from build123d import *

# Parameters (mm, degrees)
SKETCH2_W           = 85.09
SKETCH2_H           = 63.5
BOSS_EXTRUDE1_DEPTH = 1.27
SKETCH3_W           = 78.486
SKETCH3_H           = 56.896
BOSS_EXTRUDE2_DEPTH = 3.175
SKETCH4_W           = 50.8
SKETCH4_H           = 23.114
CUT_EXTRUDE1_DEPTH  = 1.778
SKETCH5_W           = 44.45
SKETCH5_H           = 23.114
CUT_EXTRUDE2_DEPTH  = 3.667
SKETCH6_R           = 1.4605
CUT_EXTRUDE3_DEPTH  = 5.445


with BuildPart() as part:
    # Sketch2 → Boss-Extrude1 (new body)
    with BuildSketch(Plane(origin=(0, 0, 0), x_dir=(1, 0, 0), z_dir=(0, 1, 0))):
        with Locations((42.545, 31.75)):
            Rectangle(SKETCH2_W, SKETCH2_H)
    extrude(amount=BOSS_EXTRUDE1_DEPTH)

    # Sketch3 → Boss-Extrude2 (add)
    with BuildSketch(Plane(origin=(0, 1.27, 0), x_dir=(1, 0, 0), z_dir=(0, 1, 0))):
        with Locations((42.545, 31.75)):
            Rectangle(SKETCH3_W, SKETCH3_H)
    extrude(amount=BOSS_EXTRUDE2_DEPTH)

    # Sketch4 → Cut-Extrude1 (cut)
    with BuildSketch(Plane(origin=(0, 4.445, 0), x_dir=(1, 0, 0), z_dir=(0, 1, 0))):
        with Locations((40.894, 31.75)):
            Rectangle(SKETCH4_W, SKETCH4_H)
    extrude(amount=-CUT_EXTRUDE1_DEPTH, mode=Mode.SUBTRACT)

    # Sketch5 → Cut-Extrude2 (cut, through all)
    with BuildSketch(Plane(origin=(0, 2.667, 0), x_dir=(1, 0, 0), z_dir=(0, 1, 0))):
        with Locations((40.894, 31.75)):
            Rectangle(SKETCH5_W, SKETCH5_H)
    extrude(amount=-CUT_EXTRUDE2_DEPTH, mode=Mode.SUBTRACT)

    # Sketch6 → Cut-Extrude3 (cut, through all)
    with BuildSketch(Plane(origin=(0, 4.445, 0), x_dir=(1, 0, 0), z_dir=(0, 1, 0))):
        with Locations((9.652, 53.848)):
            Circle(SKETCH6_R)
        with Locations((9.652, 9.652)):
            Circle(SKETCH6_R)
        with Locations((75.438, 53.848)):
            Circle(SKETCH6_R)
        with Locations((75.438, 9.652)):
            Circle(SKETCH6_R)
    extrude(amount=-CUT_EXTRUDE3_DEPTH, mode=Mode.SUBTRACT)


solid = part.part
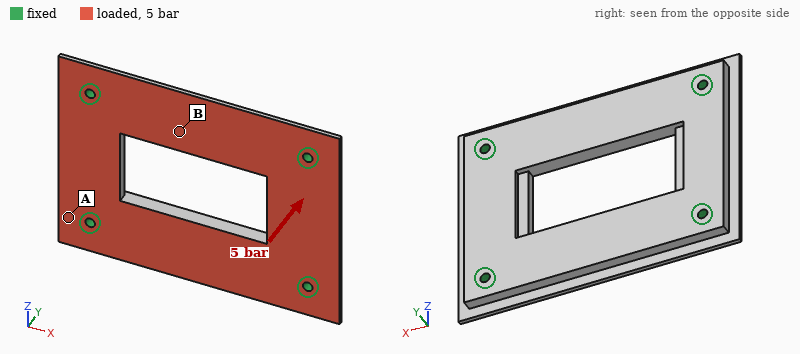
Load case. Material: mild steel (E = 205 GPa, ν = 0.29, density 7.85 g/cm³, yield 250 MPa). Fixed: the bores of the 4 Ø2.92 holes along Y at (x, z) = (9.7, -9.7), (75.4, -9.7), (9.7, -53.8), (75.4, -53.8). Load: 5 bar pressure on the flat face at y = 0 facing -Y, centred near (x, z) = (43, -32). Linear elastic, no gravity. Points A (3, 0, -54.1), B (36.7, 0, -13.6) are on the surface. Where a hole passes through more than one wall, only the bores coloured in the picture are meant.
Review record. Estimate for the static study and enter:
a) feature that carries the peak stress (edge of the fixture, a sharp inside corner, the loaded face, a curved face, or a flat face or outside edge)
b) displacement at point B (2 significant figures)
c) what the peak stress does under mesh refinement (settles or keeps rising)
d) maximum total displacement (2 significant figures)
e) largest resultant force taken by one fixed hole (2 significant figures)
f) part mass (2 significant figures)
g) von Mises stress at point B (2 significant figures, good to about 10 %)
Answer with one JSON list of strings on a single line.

["edge of the fixture", "20 µm", "keeps rising", "23 µm", "550 N", "130 g", "28 MPa"]
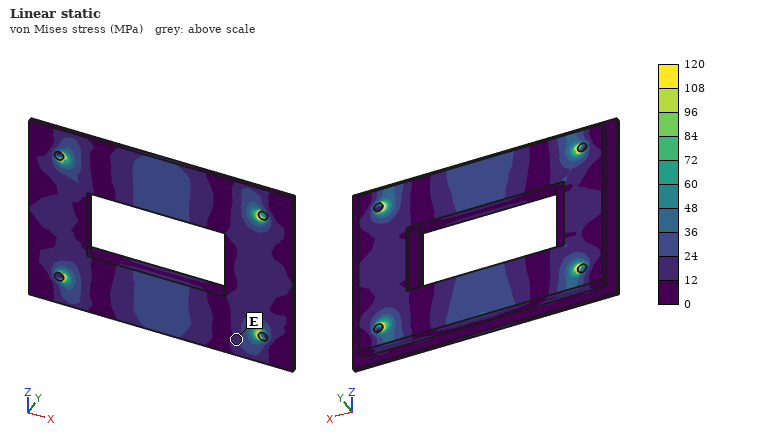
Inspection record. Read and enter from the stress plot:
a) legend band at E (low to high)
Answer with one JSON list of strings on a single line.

["12 to 24 MPa"]
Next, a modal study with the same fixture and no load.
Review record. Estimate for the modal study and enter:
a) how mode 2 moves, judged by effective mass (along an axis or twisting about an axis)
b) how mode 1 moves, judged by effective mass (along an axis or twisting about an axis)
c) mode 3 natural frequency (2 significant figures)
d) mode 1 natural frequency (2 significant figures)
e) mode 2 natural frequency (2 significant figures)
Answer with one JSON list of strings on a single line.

["twisting about X", "along Y", "9000 Hz", "4900 Hz", "5300 Hz"]
